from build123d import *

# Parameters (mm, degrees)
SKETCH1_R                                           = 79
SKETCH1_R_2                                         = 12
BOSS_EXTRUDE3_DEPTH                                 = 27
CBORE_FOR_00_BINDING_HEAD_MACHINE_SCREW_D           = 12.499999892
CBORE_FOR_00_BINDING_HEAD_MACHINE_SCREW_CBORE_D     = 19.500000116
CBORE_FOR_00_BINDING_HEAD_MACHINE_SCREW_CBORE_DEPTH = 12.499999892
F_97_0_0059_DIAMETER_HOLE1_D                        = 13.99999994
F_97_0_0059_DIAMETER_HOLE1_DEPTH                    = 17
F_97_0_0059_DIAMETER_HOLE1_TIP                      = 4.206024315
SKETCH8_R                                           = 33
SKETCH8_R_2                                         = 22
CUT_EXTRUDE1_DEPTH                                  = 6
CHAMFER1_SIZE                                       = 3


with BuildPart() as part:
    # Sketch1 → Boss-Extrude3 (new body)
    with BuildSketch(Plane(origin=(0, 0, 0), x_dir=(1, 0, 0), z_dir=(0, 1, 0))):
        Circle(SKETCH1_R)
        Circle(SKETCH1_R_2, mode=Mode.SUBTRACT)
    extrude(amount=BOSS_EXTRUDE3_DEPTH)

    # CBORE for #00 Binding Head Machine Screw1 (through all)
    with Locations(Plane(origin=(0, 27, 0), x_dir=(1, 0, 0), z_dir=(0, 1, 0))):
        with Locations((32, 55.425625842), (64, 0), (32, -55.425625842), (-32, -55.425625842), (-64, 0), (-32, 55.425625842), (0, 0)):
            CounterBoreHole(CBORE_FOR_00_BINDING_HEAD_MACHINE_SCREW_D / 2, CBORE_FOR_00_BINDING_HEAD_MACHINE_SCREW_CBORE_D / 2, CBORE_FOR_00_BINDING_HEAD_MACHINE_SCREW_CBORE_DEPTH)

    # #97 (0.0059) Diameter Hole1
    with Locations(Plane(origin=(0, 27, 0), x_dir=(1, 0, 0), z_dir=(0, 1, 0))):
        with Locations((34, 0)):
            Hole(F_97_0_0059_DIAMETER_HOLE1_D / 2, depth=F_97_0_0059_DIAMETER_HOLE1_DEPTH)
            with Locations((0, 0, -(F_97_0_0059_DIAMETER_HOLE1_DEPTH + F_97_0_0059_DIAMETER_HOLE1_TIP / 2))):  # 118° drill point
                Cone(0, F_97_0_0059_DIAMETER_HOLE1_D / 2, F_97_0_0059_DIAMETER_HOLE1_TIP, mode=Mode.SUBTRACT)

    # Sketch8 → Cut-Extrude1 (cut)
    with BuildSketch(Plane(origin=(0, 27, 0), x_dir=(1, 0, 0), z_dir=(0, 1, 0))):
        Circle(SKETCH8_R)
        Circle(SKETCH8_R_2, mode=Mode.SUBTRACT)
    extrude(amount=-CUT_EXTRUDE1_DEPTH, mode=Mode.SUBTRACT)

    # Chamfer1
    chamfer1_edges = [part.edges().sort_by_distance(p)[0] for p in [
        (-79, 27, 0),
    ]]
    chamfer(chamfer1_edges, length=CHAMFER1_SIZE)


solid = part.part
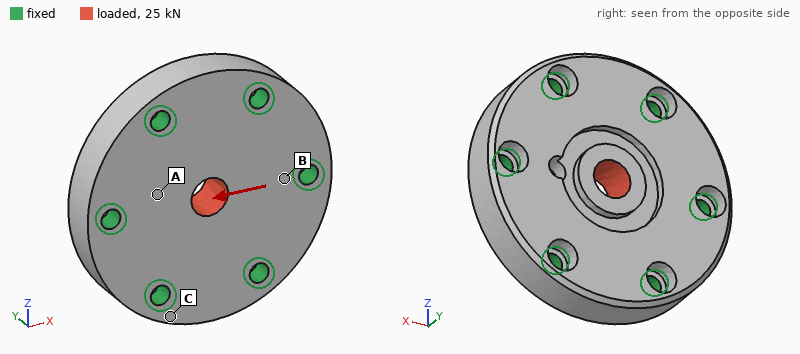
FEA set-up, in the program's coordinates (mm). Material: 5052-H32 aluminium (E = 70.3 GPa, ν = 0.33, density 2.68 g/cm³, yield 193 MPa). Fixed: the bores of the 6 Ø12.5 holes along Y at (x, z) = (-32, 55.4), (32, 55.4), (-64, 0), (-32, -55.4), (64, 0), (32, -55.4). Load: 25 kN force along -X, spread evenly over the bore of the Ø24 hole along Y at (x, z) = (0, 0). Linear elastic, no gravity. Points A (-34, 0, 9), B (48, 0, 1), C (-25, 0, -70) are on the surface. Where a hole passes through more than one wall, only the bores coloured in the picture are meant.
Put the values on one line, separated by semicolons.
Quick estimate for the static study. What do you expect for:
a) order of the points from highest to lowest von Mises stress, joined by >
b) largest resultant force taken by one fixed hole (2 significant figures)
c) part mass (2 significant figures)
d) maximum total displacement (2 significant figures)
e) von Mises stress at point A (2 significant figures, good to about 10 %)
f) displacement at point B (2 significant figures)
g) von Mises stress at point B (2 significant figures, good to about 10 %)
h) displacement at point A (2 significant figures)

B > A > C; 6.3 kN; 1.3 kg; 12 µm; 8.7 MPa; 2.0 µm; 14 MPa; 4.4 µm
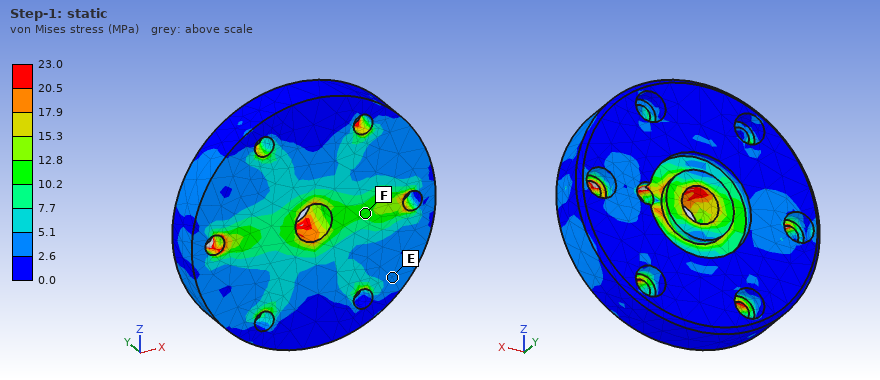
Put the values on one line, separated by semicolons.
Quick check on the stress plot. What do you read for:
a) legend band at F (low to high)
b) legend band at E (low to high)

10.2 to 12.8 MPa; 2.6 to 5.1 MPa
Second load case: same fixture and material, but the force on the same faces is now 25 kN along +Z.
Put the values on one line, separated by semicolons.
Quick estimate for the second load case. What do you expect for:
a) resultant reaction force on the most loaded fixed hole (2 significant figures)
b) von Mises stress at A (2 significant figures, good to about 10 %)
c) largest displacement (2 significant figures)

5.6 kN; 2.8 MPa; 11 µm
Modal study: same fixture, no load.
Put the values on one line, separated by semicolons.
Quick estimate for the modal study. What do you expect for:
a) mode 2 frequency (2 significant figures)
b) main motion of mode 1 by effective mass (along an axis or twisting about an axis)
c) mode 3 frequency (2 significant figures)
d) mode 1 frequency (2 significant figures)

14 kHz; along Y; 14 kHz; 8700 Hz
